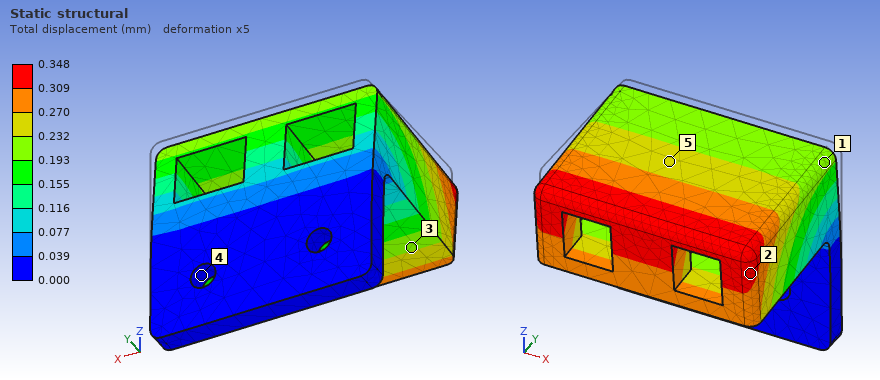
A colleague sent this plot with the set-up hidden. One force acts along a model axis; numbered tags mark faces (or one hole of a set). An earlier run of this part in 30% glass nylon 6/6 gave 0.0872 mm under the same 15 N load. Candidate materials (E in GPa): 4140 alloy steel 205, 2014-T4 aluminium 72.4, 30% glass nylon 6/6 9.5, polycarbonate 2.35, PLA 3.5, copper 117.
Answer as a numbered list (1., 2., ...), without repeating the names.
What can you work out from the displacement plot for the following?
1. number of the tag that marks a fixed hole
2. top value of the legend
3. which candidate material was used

1. 4
2. 0.348 mm
3. polycarbonate
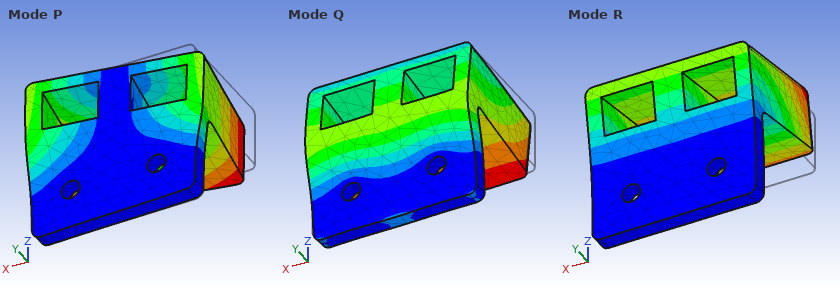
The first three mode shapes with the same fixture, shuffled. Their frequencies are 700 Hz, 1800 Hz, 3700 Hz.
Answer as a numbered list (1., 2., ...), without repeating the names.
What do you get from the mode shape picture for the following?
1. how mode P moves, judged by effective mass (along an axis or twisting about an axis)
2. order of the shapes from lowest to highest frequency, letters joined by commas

1. along X
2. R, P, Q
